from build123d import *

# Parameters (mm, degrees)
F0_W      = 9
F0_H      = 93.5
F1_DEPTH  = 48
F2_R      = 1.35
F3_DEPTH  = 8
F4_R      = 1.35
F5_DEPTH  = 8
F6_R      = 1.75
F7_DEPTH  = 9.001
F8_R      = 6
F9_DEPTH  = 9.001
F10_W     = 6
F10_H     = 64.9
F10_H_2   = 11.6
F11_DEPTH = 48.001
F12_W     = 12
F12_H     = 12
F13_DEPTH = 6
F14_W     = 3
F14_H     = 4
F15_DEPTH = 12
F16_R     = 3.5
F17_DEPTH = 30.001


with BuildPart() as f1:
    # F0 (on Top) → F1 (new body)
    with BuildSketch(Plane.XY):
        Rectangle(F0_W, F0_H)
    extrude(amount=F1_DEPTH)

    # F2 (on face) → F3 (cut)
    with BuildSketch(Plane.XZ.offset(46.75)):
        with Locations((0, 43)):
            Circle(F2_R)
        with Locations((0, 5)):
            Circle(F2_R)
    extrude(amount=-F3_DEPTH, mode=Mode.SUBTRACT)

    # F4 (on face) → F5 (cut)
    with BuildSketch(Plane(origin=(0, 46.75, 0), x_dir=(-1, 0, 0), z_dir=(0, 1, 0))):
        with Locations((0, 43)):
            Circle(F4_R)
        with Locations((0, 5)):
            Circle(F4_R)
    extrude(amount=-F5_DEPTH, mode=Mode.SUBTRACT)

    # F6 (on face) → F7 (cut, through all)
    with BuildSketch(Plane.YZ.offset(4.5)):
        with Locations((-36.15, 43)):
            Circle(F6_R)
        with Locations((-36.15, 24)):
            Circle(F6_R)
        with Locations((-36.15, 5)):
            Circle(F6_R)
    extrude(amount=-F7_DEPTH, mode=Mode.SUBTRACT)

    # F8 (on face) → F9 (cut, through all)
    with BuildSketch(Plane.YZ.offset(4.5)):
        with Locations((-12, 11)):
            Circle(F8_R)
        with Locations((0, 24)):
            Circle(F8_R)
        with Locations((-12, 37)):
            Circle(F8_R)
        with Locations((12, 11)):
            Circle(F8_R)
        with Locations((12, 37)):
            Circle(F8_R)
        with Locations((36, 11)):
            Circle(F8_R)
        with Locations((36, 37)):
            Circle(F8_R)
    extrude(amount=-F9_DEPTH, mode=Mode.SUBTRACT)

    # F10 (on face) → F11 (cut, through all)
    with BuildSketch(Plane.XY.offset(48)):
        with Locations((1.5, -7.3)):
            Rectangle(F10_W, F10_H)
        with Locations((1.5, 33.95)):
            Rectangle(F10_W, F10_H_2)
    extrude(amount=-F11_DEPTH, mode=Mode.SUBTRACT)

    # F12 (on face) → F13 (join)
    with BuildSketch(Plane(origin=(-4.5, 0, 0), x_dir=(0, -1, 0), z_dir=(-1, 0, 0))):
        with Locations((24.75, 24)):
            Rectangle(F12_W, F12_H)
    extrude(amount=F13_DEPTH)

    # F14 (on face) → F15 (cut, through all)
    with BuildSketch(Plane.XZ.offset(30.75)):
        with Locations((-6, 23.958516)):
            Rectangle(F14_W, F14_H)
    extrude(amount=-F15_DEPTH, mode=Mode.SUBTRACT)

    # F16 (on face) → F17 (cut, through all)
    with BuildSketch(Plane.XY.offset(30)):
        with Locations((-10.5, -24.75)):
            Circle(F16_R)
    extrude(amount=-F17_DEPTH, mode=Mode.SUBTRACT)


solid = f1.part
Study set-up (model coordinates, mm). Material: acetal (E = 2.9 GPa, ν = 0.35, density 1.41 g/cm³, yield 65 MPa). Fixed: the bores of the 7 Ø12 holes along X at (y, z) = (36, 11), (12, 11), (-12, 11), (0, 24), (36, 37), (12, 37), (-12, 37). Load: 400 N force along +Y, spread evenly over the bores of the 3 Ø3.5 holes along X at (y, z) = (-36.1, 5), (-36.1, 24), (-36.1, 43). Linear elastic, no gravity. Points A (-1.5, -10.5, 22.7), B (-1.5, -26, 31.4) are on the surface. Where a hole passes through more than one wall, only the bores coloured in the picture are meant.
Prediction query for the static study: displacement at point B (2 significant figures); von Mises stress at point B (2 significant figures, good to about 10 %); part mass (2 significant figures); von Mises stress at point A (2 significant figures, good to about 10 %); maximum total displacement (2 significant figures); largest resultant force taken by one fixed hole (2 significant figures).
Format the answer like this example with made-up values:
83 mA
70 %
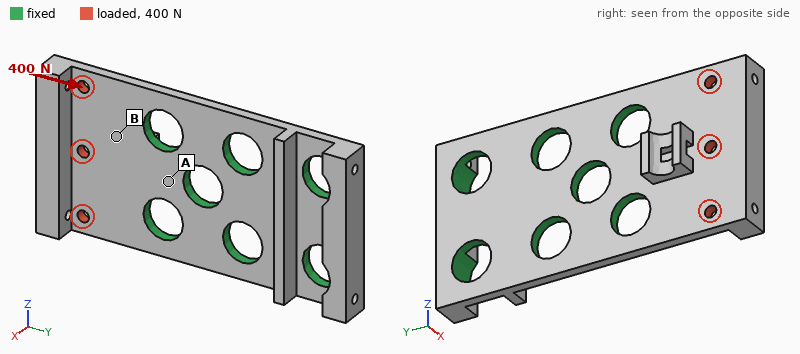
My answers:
9.5 µm
2.8 MPa
23 g
1.1 MPa
36 µm
180 N
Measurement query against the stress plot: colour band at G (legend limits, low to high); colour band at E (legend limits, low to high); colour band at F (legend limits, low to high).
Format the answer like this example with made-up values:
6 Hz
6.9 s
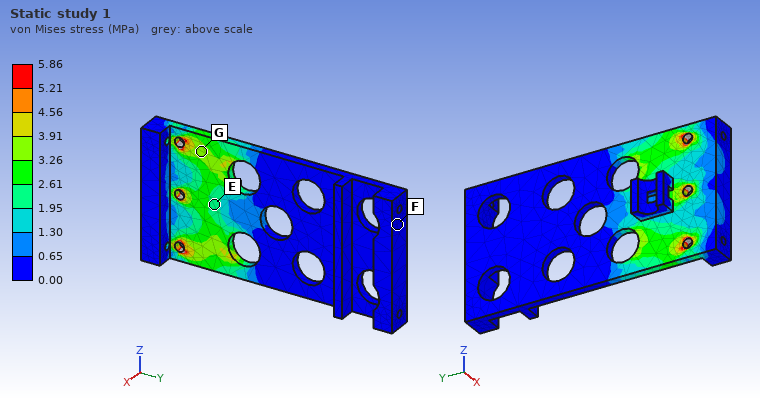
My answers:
3.26 to 3.91 MPa
1.95 to 2.61 MPa
0.00 to 0.65 MPa
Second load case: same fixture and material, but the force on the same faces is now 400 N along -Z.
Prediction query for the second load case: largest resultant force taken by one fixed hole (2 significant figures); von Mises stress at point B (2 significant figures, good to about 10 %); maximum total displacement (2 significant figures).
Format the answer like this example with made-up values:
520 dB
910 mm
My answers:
310 N
6.7 MPa
0.11 mm
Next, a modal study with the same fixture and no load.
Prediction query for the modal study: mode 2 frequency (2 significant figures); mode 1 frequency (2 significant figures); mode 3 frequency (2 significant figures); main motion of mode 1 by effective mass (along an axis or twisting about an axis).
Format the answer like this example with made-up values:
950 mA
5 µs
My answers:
1200 Hz
560 Hz
3000 Hz
along X
